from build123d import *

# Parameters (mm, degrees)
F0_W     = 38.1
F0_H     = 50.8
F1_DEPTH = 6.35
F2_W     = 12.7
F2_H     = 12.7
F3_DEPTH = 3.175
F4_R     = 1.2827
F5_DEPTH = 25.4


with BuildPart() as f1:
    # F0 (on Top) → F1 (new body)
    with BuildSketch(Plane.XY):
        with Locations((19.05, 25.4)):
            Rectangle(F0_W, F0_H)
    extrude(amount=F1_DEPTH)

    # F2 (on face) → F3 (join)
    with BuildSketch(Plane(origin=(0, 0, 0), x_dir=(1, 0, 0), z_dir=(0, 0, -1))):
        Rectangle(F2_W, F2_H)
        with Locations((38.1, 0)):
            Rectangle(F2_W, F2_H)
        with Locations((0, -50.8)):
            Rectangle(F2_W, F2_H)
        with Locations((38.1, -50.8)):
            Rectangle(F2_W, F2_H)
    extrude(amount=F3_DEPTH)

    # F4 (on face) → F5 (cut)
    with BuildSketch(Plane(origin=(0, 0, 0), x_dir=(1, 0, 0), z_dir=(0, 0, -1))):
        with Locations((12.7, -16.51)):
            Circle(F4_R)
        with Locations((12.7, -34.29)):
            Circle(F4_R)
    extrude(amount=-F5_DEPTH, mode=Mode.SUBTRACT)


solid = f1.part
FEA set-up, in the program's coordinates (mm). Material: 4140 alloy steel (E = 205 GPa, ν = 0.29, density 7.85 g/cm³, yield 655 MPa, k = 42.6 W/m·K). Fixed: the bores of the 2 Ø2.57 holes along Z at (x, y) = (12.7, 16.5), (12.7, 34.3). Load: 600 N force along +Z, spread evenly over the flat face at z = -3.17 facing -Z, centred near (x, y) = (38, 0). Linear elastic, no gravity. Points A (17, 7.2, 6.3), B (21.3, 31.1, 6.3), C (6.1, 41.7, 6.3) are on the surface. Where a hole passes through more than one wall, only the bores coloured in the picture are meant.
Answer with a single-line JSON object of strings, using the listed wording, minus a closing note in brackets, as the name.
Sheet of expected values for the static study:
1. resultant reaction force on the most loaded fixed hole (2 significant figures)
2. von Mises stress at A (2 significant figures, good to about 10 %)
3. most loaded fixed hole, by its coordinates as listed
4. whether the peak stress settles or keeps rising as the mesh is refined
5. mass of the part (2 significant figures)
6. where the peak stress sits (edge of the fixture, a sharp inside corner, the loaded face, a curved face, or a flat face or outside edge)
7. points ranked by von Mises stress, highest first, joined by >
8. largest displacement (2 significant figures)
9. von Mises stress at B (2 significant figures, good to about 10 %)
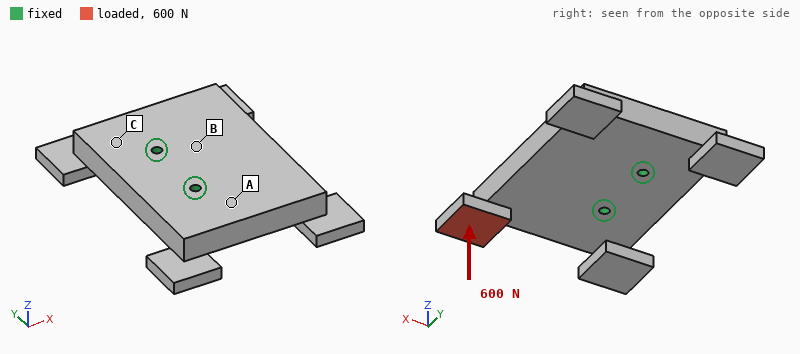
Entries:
{"resultant reaction force on the most loaded fixed hole": "890 N", "von Mises stress at A": "56 MPa", "most loaded fixed hole, by its coordinates as listed": "(12.7, 16.5)", "whether the peak stress settles or keeps rising as the mesh is refined": "keeps rising", "mass of the part": "110 g", "where the peak stress sits": "edge of the fixture", "points ranked by von Mises stress, highest first, joined by >": "A > B > C", "largest displacement": "96 µm", "von Mises stress at B": "31 MPa"}
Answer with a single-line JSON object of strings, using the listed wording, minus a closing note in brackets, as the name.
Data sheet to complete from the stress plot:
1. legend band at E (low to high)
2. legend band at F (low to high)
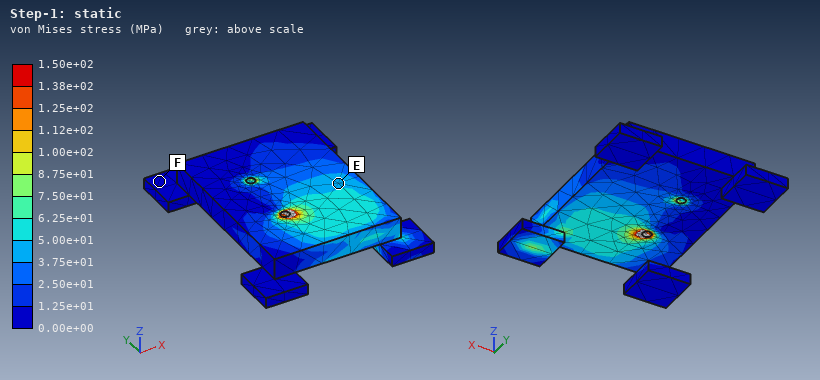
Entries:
{"legend band at E": "3.75e+01 to 5.00e+01 MPa", "legend band at F": "0.00e+00 to 1.25e+01 MPa"}
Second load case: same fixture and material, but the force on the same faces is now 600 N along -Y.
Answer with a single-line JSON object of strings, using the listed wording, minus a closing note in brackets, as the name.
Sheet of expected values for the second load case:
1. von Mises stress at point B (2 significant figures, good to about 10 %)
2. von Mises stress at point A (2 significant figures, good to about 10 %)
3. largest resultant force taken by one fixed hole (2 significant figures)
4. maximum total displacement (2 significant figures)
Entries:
{"von Mises stress at point B": "8.3 MPa", "von Mises stress at point A": "16 MPa", "largest resultant force taken by one fixed hole": "870 N", "maximum total displacement": "27 µm"}
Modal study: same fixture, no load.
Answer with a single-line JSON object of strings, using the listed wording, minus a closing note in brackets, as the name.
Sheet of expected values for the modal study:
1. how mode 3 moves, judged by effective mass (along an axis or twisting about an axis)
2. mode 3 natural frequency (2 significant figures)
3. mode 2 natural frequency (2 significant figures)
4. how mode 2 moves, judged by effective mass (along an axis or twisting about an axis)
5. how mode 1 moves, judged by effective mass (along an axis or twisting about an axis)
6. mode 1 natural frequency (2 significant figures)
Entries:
{"how mode 3 moves, judged by effective mass": "along Z", "mode 3 natural frequency": "8800 Hz", "mode 2 natural frequency": "5800 Hz", "how mode 2 moves, judged by effective mass": "twisting about X", "how mode 1 moves, judged by effective mass": "along Z", "mode 1 natural frequency": "4800 Hz"}
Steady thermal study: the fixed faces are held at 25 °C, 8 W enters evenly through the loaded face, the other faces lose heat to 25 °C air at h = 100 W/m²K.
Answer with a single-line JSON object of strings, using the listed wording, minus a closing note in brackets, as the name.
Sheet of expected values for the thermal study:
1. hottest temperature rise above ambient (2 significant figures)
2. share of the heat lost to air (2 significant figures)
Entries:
{"hottest temperature rise above ambient": "53 K", "share of the heat lost to air": "48 %"}
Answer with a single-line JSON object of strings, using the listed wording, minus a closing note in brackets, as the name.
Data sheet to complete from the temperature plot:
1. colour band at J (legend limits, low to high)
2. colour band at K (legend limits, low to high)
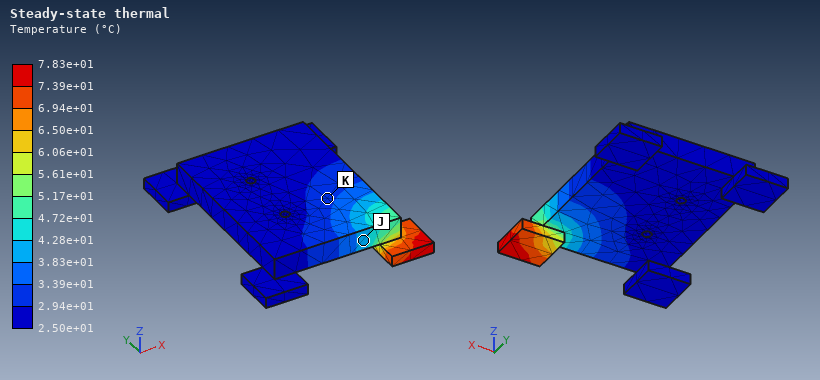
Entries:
{"colour band at J": "3.83e+01 to 4.28e+01 °C", "colour band at K": "2.94e+01 to 3.39e+01 °C"}
